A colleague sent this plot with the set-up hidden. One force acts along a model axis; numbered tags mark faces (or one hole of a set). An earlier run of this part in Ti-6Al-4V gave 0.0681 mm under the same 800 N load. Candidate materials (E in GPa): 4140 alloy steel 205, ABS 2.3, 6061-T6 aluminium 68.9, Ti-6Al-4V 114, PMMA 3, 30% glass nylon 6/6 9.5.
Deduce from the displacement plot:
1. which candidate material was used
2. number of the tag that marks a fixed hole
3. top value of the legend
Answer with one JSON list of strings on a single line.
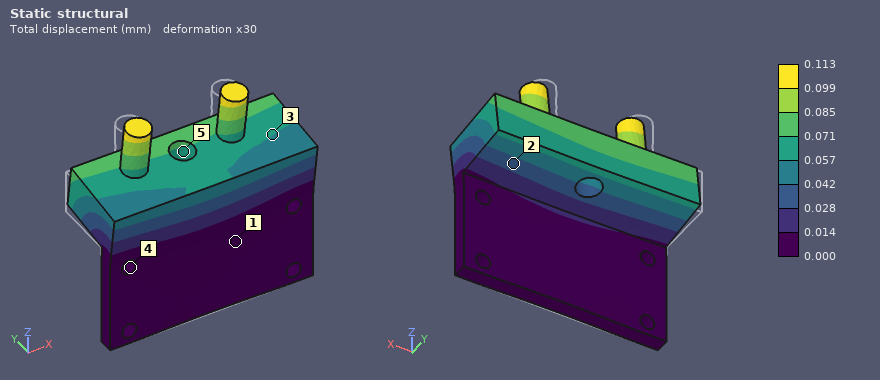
["6061-T6 aluminium", "4", "0.113 mm"]
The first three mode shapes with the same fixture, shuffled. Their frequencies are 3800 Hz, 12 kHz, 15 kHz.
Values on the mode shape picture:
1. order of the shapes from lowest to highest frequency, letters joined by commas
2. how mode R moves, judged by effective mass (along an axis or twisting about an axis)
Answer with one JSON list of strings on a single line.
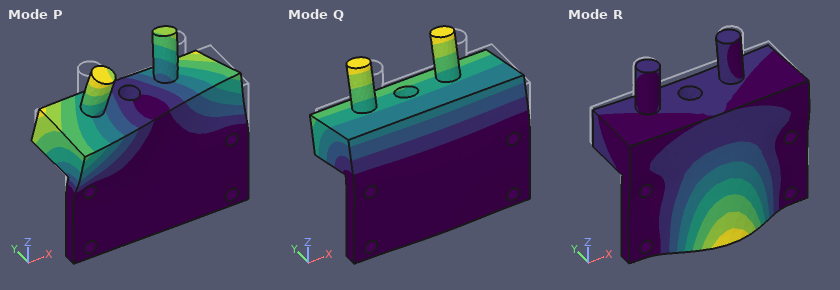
["Q, P, R", "along Y"]
